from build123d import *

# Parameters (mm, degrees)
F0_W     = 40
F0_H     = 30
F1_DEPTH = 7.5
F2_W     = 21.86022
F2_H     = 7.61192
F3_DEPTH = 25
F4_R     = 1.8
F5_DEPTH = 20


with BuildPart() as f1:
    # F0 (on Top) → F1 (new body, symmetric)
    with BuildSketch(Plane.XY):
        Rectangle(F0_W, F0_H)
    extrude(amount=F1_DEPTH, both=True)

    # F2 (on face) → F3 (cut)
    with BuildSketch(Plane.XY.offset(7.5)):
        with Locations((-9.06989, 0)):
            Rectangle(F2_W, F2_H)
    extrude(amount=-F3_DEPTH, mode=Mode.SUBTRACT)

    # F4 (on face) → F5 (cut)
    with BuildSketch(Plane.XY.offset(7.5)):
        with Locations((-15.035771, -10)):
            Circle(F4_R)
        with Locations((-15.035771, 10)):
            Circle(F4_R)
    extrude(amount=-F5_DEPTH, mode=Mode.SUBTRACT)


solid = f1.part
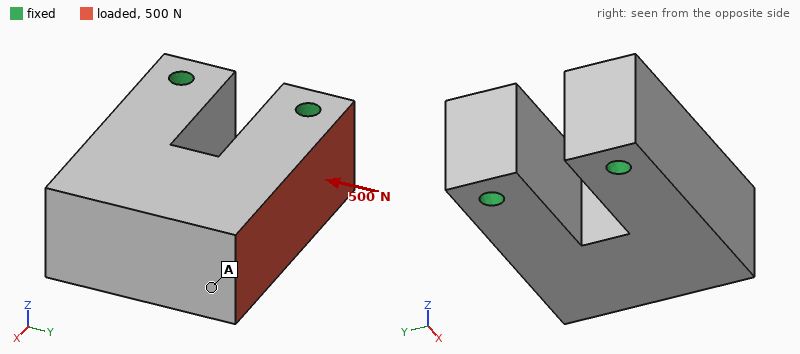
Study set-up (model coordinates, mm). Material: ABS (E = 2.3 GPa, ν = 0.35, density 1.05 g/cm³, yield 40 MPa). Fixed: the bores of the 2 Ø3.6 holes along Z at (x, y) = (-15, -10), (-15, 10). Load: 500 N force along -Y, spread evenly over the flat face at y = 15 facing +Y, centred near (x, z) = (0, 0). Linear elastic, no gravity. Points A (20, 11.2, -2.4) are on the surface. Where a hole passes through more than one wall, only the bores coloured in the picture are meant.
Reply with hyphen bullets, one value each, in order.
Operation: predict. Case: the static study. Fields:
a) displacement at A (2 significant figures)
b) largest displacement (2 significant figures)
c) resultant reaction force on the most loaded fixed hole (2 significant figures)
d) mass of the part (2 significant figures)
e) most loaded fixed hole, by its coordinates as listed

- 0.11 mm
- 0.11 mm
- 420 N
- 16 g
- (-15, 10)
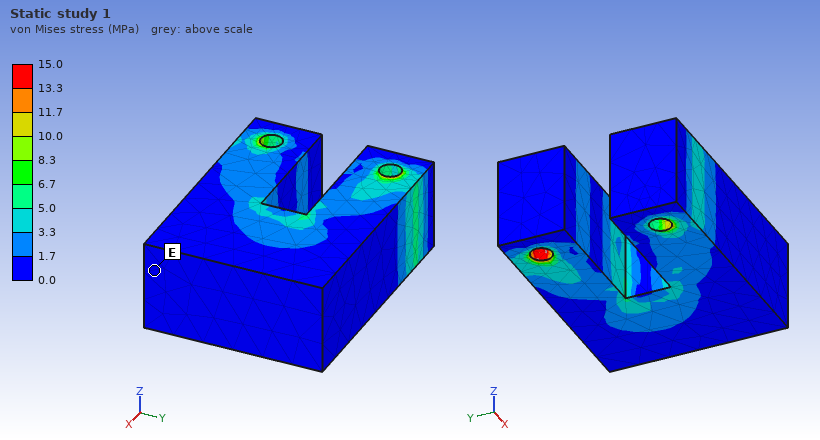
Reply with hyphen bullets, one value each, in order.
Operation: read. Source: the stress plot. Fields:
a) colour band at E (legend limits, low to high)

- 0.0 to 1.7 MPa
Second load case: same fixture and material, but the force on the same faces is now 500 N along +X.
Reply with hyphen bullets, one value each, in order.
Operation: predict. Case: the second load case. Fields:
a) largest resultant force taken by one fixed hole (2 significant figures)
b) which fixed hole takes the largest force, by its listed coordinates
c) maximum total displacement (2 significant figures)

- 570 N
- (-15, 10)
- 70 µm
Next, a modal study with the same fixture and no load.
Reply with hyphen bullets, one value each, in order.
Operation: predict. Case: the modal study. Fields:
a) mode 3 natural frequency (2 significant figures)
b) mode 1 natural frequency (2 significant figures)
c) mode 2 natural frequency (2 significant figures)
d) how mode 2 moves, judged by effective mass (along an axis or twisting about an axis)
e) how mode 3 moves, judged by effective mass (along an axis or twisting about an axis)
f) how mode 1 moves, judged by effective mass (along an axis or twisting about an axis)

- 4400 Hz
- 2200 Hz
- 2900 Hz
- along Y
- twisting about X
- along Z
